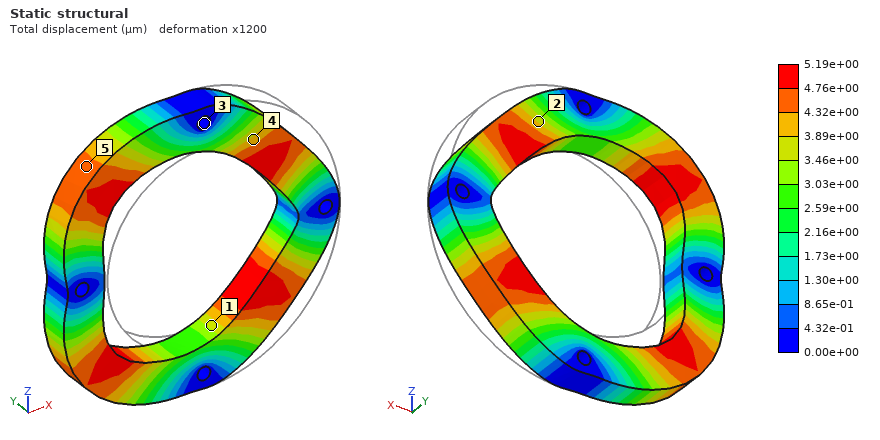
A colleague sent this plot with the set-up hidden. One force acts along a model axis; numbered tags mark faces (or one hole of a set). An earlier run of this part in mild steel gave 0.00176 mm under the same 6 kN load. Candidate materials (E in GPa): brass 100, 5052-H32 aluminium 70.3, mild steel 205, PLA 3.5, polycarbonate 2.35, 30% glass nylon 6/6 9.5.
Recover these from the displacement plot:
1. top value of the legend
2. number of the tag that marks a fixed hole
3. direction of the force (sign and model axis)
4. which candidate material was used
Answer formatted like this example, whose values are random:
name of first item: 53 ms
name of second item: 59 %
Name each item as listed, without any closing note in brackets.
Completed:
top value of the legend: 5.19e+00 µm
number of the tag that marks a fixed hole: 3
direction of the force: -X
which candidate material was used: 5052-H32 aluminium
